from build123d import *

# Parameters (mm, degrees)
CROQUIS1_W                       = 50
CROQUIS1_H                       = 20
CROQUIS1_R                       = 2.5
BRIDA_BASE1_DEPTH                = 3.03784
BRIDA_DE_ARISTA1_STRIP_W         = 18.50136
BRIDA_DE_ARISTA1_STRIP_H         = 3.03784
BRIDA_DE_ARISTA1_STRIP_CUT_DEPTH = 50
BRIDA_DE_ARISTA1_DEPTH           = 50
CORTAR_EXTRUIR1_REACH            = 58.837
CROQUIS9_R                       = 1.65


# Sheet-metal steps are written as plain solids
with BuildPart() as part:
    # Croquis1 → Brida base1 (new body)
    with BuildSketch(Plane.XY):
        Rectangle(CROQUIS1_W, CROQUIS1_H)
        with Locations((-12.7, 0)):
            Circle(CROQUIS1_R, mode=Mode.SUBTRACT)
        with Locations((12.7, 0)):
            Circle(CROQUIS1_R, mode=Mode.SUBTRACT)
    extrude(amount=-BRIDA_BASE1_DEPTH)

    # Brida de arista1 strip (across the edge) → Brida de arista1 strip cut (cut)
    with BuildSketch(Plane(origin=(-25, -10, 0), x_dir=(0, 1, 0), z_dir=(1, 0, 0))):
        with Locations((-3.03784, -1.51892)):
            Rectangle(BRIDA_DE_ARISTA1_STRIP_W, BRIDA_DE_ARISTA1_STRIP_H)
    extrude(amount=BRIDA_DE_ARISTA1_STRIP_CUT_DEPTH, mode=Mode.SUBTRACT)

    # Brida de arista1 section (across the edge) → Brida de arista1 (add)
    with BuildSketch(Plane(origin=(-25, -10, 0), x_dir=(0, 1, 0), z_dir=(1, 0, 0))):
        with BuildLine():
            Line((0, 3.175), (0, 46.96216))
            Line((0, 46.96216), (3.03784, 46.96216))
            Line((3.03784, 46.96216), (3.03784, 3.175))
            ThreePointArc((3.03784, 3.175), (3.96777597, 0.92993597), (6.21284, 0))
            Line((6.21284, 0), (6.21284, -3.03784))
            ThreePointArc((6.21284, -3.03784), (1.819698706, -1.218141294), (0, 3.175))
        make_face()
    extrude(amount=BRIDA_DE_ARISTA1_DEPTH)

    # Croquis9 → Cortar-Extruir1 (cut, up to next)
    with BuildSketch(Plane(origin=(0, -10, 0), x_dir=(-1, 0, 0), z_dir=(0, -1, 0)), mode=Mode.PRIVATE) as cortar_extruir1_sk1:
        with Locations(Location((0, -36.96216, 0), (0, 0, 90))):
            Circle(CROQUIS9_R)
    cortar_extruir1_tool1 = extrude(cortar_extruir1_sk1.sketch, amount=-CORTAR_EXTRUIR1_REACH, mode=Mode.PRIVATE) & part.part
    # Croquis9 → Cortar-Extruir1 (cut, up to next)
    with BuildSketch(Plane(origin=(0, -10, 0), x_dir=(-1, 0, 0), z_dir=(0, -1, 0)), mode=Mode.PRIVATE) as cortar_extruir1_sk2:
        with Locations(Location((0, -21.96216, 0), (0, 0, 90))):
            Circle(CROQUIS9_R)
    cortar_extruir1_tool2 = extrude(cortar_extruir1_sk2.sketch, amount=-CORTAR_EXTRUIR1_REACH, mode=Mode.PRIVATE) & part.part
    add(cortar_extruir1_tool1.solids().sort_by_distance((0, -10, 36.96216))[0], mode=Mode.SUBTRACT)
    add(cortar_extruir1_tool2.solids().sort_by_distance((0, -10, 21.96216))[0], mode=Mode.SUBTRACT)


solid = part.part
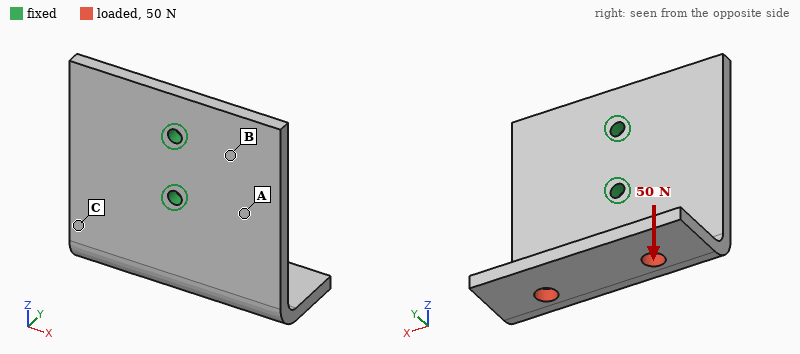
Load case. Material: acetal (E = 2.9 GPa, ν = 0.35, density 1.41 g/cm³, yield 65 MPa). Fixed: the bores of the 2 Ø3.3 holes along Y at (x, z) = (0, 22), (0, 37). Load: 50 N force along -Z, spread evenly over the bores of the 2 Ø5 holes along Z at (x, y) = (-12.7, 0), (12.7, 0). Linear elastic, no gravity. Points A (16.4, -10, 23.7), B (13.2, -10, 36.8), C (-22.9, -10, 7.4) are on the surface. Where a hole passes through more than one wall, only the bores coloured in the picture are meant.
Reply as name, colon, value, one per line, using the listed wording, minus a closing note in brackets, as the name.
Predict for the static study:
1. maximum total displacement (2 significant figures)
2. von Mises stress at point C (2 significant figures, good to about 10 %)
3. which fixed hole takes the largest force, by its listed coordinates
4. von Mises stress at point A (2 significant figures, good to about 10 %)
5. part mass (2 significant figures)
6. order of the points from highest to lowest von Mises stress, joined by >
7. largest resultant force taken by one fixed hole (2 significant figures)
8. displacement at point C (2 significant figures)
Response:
maximum total displacement: 0.76 mm
von Mises stress at point C: 5.1 MPa
which fixed hole takes the largest force, by its listed coordinates: (0, 22)
von Mises stress at point A: 2.9 MPa
part mass: 14 g
order of the points from highest to lowest von Mises stress, joined by >: C > A > B
largest resultant force taken by one fixed hole: 38 N
displacement at point C: 0.17 mm
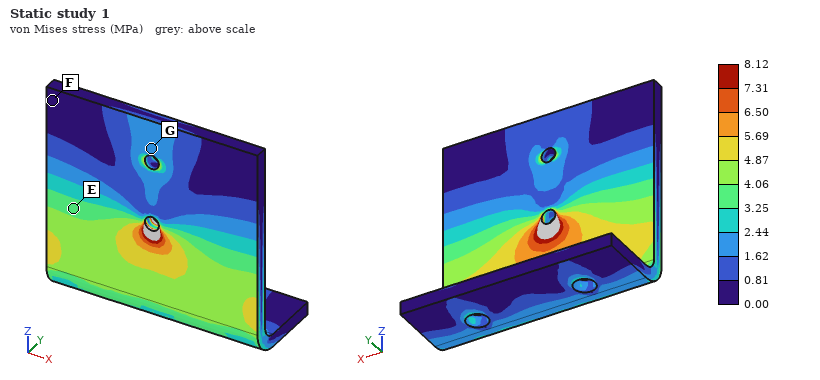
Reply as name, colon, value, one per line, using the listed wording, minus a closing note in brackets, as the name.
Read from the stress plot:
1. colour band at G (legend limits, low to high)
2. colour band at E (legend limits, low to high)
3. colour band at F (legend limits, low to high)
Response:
colour band at G: 1.62 to 2.44 MPa
colour band at E: 3.25 to 4.06 MPa
colour band at F: 0.00 to 0.81 MPa
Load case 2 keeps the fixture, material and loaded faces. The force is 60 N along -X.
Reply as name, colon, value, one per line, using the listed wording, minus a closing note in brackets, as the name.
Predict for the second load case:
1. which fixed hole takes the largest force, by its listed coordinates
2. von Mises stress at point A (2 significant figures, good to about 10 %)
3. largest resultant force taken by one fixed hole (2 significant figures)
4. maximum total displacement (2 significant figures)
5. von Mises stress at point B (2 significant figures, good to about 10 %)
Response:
which fixed hole takes the largest force, by its listed coordinates: (0, 22)
von Mises stress at point A: 3.9 MPa
largest resultant force taken by one fixed hole: 140 N
maximum total displacement: 0.79 mm
von Mises stress at point B: 2.9 MPa
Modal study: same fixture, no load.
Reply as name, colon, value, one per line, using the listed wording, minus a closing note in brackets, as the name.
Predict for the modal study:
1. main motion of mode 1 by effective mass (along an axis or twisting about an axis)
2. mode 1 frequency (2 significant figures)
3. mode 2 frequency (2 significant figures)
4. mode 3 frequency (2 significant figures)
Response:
main motion of mode 1 by effective mass: along Y
mode 1 frequency: 480 Hz
mode 2 frequency: 540 Hz
mode 3 frequency: 1300 Hz
